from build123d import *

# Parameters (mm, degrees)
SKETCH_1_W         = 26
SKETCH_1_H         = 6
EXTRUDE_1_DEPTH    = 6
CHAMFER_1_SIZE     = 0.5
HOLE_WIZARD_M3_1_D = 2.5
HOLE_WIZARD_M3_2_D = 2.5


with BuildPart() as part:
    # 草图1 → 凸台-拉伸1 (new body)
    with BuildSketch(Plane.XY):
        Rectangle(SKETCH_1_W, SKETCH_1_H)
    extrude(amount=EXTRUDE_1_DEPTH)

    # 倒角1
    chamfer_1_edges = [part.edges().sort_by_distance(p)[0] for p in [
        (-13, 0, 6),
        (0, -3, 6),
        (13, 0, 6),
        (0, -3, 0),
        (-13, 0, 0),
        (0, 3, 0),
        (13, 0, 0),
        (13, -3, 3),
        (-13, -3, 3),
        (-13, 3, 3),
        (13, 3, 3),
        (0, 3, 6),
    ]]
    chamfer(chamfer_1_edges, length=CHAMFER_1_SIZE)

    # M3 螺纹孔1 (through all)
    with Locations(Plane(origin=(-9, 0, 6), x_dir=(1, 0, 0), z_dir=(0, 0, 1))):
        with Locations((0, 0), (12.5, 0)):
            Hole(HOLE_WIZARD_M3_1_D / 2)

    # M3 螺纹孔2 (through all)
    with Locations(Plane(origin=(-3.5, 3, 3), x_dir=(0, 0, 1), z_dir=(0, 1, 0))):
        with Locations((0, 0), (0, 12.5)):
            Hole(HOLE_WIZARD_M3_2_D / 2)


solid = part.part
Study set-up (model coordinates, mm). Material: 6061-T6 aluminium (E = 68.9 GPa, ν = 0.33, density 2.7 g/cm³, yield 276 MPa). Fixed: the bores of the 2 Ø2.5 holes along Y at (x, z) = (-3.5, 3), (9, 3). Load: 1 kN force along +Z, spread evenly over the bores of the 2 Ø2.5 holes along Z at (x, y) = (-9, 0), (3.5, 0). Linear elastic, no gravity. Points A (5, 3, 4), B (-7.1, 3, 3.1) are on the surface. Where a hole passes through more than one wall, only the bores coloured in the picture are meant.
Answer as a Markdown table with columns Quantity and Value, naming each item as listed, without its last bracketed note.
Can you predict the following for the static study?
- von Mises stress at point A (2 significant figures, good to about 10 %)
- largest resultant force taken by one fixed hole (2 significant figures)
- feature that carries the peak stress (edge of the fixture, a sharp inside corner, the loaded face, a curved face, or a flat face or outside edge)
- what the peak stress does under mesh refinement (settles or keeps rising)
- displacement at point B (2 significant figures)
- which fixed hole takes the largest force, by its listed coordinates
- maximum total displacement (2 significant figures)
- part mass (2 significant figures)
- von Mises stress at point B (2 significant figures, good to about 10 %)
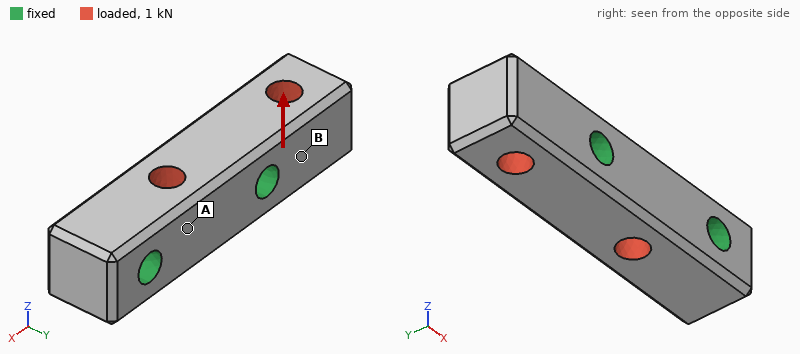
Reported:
| Quantity | Value |
|---|---|
| von Mises stress at point A | 11 MPa |
| largest resultant force taken by one fixed hole | 770 N |
| feature that carries the peak stress | edge of the fixture |
| what the peak stress does under mesh refinement | keeps rising |
| displacement at point B | 4.0 µm |
| which fixed hole takes the largest force, by its listed coordinates | (-3.5, 3) |
| maximum total displacement | 15 µm |
| part mass | 2.2 g |
| von Mises stress at point B | 33 MPa |
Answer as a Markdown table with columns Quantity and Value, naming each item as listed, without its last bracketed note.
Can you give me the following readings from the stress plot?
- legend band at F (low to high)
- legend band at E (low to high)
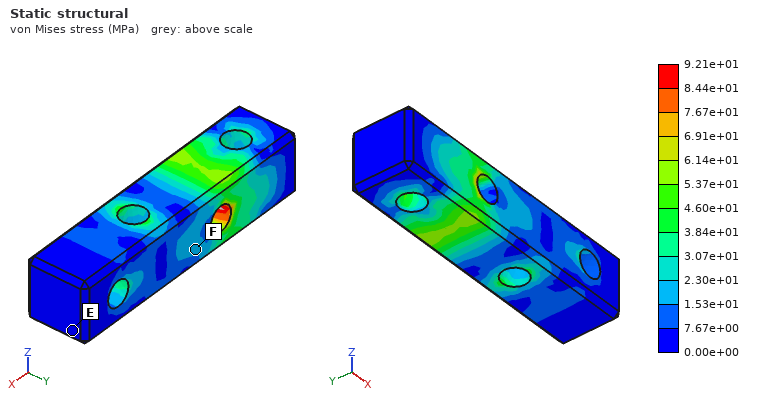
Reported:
| Quantity | Value |
|---|---|
| legend band at F | 1.53e+01 to 2.30e+01 MPa |
| legend band at E | 0.00e+00 to 7.67e+00 MPa |
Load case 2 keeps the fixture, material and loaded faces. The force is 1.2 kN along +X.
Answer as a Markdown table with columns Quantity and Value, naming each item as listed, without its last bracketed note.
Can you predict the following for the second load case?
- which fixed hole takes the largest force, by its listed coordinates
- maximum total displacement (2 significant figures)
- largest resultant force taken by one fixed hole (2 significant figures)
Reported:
| Quantity | Value |
|---|---|
| which fixed hole takes the largest force, by its listed coordinates | (-3.5, 3) |
| maximum total displacement | 2.2 µm |
| largest resultant force taken by one fixed hole | 850 N |
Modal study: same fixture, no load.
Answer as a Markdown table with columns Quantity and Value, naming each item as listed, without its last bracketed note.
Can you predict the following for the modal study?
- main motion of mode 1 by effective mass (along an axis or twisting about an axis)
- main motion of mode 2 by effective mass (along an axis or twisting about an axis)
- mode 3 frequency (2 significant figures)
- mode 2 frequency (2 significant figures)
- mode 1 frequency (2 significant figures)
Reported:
| Quantity | Value |
|---|---|
| main motion of mode 1 by effective mass | along Z |
| main motion of mode 2 by effective mass | along Y |
| mode 3 frequency | 76 kHz |
| mode 2 frequency | 45 kHz |
| mode 1 frequency | 39 kHz |
